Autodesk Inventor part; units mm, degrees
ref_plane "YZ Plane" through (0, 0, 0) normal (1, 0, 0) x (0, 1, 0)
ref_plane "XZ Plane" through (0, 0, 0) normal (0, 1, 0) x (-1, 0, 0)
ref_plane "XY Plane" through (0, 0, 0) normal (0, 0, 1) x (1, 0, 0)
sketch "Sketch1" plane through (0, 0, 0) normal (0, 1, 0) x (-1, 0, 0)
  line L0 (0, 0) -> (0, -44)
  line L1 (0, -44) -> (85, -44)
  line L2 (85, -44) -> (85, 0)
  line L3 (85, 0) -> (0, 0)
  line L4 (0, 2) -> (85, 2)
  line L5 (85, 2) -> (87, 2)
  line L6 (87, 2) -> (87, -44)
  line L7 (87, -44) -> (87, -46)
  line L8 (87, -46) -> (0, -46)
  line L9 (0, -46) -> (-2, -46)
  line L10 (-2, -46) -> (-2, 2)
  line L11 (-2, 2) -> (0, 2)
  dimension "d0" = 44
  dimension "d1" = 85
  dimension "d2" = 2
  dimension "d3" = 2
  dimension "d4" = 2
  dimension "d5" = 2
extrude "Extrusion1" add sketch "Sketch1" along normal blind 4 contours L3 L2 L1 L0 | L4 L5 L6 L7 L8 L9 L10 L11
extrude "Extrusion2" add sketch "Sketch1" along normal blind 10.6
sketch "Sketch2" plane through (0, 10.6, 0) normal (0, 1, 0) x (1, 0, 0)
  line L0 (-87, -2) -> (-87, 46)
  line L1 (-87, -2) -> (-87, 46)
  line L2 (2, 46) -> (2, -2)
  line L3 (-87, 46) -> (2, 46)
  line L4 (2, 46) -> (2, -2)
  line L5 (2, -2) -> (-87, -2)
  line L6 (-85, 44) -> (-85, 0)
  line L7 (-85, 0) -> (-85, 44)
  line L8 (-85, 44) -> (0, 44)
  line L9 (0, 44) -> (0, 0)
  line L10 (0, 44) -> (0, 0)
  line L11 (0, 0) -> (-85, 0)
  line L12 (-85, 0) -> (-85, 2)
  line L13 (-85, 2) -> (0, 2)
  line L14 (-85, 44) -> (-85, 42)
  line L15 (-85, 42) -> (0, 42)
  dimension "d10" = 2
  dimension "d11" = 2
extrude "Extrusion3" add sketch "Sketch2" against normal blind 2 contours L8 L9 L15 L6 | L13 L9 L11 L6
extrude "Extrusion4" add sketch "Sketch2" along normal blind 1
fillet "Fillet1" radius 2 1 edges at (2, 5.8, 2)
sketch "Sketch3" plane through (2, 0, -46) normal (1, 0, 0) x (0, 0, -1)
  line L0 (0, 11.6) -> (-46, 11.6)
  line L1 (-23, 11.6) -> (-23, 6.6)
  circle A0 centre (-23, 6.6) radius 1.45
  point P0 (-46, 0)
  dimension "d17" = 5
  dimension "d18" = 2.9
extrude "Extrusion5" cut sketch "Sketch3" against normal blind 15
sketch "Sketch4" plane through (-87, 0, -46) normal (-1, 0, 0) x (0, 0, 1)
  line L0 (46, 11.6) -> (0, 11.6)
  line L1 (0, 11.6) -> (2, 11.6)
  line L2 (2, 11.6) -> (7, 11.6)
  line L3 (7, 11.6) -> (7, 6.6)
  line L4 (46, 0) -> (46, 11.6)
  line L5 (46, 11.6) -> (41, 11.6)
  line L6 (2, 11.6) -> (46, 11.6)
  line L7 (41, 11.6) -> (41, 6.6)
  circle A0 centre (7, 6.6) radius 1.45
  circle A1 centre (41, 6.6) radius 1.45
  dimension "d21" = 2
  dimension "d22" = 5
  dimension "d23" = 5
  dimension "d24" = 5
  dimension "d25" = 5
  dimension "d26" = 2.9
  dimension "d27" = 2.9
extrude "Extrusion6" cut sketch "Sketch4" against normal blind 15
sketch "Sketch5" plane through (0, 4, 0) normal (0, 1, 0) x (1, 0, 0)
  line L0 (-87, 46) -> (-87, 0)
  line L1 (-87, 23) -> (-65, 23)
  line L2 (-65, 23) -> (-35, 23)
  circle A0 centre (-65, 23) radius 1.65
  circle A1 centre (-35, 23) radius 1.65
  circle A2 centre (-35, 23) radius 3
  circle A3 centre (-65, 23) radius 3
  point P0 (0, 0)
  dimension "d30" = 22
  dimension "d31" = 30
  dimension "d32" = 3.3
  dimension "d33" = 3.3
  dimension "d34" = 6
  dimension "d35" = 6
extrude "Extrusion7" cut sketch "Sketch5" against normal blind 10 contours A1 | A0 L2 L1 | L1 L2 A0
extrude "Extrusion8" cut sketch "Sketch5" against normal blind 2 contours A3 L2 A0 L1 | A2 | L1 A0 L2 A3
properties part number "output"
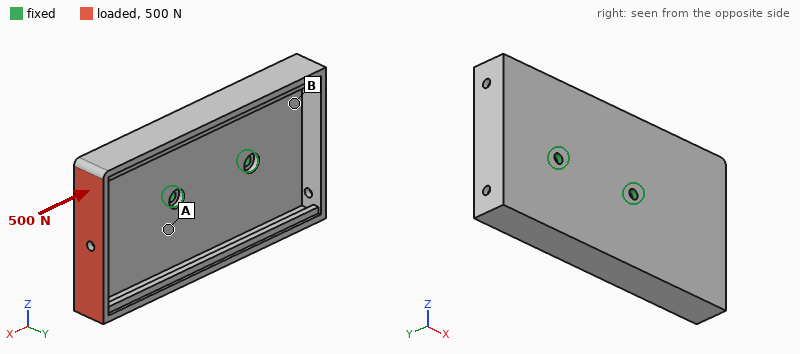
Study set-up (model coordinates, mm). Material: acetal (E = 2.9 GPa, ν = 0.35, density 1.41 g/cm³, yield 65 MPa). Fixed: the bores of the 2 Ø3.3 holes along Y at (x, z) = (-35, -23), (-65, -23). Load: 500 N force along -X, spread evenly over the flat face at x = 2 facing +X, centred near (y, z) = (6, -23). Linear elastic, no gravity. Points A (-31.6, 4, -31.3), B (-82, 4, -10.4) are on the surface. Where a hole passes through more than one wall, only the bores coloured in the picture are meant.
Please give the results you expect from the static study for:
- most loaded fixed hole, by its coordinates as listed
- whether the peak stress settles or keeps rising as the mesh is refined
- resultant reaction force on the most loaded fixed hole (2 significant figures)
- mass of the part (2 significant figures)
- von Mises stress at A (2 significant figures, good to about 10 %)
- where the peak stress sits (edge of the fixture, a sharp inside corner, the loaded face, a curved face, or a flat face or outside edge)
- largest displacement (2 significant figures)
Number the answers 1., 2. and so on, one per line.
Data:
1. (-35, -23)
2. keeps rising
3. 290 N
4. 30 g
5. 6.3 MPa
6. edge of the fixture
7. 1.1 mm
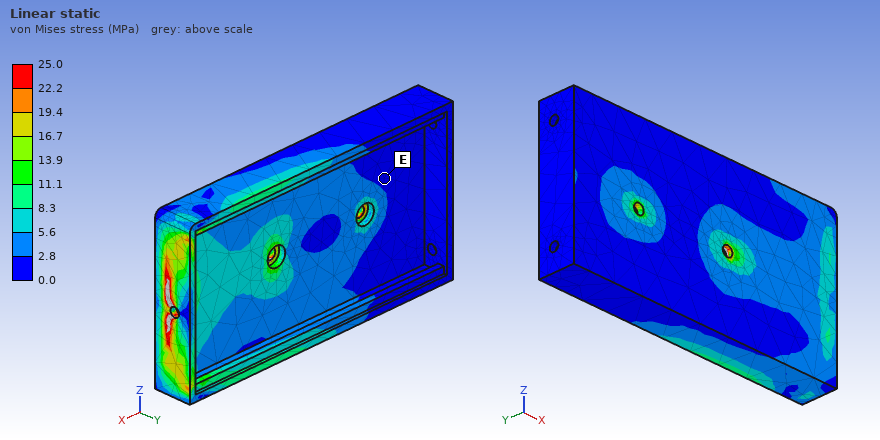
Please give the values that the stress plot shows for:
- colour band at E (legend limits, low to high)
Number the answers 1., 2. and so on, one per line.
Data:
1. 0.0 to 2.8 MPa
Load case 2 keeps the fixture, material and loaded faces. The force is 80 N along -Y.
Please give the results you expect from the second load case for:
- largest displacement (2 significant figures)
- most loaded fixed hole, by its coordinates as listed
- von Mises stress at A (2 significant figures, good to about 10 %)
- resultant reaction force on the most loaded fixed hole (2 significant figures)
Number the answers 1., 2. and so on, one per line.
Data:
1. 1.2 mm
2. (-35, -23)
3. 9.4 MPa
4. 180 N
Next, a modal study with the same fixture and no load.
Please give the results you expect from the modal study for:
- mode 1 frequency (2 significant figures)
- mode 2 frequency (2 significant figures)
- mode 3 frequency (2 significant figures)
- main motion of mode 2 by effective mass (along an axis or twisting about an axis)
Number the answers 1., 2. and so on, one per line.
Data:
1. 430 Hz
2. 580 Hz
3. 730 Hz
4. along Y
